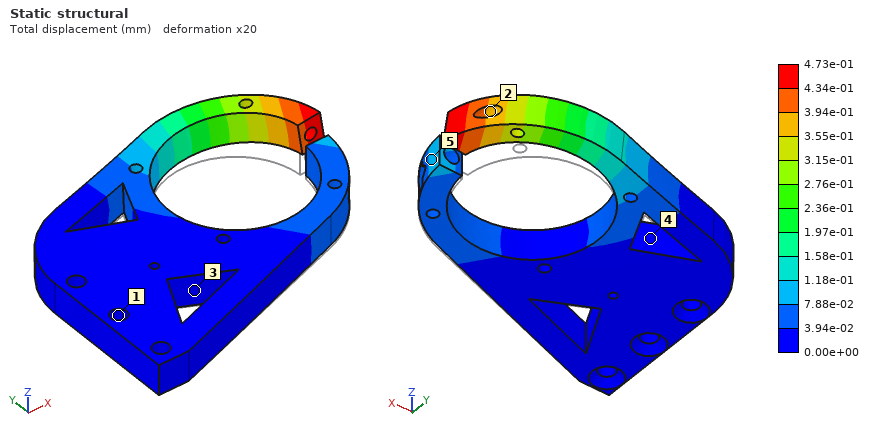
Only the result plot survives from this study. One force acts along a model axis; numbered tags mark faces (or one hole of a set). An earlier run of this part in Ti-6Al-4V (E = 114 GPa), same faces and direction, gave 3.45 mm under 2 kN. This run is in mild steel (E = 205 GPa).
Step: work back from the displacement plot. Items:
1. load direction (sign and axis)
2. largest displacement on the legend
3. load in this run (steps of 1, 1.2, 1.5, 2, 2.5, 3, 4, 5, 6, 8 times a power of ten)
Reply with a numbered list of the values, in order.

1. +Z
2. 4.73e-01 mm
3. 500 N
